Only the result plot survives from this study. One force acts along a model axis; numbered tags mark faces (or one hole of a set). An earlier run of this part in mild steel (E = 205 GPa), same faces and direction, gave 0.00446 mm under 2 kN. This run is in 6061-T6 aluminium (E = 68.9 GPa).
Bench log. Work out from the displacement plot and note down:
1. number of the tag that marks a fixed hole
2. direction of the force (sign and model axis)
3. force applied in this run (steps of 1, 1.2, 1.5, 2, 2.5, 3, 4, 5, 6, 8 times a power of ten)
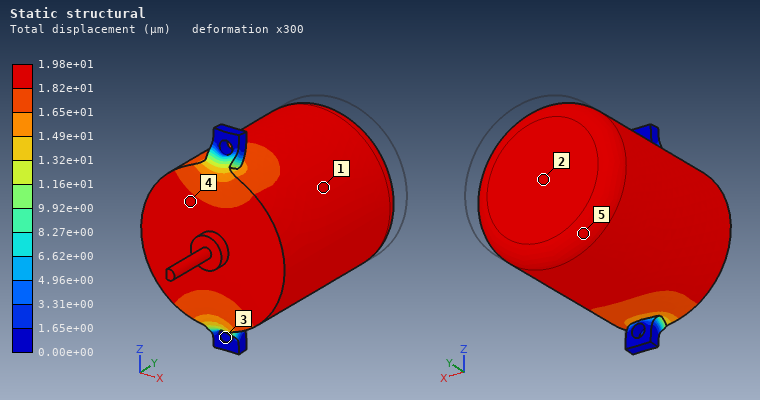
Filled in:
3
-Y
3 kN
